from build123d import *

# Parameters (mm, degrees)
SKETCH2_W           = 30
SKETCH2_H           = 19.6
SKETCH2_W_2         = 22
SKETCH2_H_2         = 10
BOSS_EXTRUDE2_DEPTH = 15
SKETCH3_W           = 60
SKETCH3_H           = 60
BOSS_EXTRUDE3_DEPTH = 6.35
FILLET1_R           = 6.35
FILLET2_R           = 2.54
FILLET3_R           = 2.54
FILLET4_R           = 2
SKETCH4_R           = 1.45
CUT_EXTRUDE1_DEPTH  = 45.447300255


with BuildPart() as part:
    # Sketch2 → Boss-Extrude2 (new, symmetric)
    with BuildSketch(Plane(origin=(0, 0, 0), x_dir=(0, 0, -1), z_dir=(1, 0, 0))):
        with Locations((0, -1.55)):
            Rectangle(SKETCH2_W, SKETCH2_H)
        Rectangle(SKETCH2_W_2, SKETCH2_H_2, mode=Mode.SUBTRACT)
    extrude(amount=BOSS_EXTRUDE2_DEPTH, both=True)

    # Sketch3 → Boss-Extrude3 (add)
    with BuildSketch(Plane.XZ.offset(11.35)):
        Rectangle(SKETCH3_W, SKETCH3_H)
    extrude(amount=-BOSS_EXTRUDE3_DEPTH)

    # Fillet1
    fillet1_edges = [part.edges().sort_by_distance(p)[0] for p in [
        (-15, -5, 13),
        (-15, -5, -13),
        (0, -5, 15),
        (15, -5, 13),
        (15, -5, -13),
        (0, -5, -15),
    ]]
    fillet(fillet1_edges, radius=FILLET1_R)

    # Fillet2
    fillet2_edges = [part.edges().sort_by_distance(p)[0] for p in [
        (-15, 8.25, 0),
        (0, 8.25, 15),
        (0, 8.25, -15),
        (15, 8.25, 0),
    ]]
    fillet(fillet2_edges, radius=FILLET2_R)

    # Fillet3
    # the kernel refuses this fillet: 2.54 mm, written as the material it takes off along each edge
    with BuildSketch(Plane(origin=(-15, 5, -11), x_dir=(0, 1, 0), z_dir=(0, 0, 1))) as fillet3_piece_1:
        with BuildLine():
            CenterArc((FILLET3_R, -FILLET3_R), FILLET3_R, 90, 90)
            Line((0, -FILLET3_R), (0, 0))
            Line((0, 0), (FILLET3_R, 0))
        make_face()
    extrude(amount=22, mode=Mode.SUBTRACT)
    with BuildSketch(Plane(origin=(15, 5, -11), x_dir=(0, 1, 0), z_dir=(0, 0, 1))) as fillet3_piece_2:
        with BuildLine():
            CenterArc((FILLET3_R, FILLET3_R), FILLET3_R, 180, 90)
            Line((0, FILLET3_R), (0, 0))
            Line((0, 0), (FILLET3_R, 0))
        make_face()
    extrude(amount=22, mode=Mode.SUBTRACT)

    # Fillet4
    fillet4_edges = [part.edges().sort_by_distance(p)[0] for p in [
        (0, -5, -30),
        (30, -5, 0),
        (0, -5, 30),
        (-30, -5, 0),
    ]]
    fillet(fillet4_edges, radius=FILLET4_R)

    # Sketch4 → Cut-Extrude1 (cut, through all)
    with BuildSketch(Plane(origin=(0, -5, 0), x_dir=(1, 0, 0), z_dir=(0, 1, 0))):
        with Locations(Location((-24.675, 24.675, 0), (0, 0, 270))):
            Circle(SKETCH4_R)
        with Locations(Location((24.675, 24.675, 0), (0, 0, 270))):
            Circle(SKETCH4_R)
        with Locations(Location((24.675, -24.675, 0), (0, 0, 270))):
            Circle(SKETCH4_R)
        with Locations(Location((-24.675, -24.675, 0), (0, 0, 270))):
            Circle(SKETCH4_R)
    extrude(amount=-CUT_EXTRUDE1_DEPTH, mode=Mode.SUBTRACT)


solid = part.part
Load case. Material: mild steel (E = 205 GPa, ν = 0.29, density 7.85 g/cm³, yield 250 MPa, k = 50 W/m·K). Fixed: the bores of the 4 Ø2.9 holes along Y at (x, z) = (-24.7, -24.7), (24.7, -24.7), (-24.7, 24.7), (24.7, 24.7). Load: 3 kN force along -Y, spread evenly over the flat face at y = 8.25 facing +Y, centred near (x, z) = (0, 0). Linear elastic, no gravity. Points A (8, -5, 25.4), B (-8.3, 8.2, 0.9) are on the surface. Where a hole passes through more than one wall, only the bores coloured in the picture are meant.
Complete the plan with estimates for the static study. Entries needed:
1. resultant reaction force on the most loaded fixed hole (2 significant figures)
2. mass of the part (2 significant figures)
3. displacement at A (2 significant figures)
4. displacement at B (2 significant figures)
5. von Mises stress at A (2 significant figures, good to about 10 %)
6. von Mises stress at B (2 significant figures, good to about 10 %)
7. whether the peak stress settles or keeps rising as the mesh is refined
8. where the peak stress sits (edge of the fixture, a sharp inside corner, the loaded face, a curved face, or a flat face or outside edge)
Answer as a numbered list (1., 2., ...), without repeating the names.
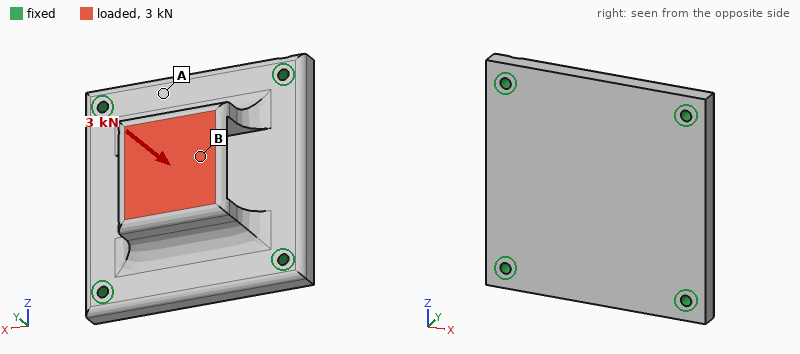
1. 810 N
2. 220 g
3. 4.9 µm
4. 16 µm
5. 14 MPa
6. 71 MPa
7. keeps rising
8. edge of the fixture
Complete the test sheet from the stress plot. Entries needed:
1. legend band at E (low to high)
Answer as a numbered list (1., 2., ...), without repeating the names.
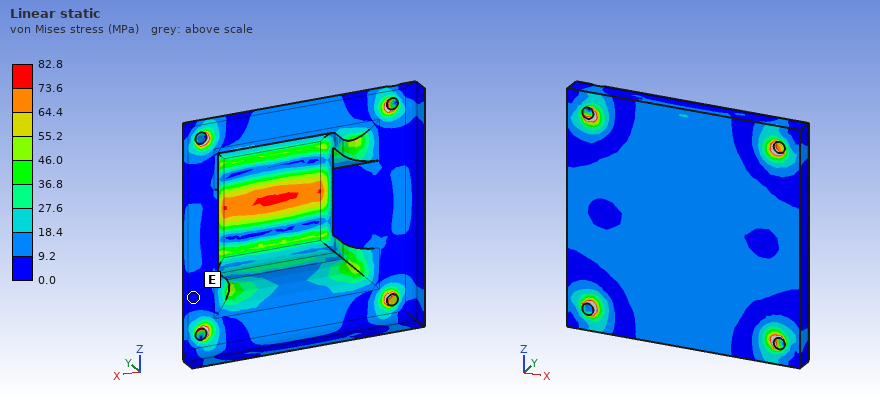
1. 0.0 to 9.2 MPa
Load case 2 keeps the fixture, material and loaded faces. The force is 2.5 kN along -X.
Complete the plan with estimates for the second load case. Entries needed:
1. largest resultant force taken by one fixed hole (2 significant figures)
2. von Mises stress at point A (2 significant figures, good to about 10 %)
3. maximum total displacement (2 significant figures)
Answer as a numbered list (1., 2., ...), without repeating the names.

1. 820 N
2. 11 MPa
3. 7.6 µm
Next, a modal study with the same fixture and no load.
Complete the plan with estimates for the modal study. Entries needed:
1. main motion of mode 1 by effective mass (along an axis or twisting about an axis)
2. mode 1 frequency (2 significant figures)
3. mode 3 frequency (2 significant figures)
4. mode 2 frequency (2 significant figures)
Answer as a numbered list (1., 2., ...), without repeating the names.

1. along Y
2. 8200 Hz
3. 13 kHz
4. 12 kHz
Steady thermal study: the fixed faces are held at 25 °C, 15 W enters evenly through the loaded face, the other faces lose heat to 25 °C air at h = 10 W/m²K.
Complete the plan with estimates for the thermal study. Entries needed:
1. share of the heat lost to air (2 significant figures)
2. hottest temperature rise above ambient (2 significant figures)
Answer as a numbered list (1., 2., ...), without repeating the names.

1. 7.0 %
2. 33 K
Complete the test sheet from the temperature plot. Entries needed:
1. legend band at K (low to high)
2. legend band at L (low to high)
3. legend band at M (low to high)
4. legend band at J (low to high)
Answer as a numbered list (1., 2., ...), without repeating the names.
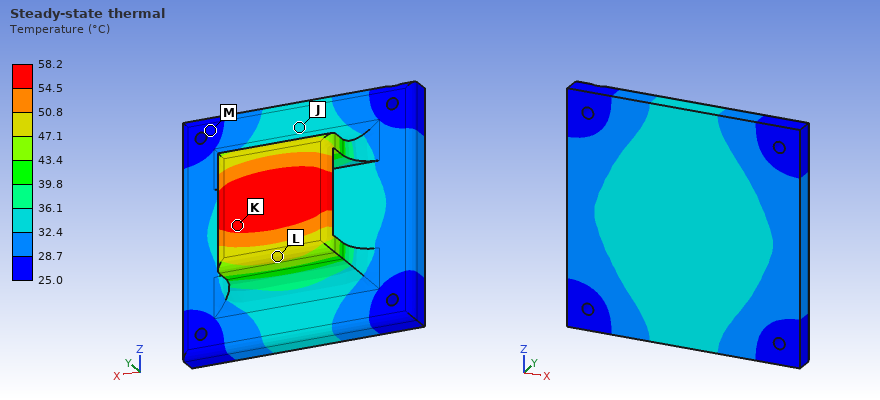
1. 54.5 to 58.2 °C
2. 47.1 to 50.8 °C
3. 25.0 to 28.7 °C
4. 32.4 to 36.1 °C
